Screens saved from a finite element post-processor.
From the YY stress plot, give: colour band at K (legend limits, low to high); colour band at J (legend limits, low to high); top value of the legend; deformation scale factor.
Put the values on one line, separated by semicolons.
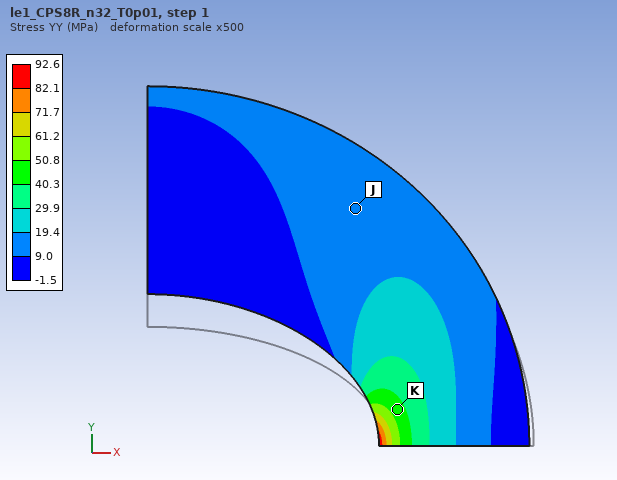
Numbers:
40.3 to 50.8 MPa; 9.0 to 19.4 MPa; 92.6 MPa; 500
